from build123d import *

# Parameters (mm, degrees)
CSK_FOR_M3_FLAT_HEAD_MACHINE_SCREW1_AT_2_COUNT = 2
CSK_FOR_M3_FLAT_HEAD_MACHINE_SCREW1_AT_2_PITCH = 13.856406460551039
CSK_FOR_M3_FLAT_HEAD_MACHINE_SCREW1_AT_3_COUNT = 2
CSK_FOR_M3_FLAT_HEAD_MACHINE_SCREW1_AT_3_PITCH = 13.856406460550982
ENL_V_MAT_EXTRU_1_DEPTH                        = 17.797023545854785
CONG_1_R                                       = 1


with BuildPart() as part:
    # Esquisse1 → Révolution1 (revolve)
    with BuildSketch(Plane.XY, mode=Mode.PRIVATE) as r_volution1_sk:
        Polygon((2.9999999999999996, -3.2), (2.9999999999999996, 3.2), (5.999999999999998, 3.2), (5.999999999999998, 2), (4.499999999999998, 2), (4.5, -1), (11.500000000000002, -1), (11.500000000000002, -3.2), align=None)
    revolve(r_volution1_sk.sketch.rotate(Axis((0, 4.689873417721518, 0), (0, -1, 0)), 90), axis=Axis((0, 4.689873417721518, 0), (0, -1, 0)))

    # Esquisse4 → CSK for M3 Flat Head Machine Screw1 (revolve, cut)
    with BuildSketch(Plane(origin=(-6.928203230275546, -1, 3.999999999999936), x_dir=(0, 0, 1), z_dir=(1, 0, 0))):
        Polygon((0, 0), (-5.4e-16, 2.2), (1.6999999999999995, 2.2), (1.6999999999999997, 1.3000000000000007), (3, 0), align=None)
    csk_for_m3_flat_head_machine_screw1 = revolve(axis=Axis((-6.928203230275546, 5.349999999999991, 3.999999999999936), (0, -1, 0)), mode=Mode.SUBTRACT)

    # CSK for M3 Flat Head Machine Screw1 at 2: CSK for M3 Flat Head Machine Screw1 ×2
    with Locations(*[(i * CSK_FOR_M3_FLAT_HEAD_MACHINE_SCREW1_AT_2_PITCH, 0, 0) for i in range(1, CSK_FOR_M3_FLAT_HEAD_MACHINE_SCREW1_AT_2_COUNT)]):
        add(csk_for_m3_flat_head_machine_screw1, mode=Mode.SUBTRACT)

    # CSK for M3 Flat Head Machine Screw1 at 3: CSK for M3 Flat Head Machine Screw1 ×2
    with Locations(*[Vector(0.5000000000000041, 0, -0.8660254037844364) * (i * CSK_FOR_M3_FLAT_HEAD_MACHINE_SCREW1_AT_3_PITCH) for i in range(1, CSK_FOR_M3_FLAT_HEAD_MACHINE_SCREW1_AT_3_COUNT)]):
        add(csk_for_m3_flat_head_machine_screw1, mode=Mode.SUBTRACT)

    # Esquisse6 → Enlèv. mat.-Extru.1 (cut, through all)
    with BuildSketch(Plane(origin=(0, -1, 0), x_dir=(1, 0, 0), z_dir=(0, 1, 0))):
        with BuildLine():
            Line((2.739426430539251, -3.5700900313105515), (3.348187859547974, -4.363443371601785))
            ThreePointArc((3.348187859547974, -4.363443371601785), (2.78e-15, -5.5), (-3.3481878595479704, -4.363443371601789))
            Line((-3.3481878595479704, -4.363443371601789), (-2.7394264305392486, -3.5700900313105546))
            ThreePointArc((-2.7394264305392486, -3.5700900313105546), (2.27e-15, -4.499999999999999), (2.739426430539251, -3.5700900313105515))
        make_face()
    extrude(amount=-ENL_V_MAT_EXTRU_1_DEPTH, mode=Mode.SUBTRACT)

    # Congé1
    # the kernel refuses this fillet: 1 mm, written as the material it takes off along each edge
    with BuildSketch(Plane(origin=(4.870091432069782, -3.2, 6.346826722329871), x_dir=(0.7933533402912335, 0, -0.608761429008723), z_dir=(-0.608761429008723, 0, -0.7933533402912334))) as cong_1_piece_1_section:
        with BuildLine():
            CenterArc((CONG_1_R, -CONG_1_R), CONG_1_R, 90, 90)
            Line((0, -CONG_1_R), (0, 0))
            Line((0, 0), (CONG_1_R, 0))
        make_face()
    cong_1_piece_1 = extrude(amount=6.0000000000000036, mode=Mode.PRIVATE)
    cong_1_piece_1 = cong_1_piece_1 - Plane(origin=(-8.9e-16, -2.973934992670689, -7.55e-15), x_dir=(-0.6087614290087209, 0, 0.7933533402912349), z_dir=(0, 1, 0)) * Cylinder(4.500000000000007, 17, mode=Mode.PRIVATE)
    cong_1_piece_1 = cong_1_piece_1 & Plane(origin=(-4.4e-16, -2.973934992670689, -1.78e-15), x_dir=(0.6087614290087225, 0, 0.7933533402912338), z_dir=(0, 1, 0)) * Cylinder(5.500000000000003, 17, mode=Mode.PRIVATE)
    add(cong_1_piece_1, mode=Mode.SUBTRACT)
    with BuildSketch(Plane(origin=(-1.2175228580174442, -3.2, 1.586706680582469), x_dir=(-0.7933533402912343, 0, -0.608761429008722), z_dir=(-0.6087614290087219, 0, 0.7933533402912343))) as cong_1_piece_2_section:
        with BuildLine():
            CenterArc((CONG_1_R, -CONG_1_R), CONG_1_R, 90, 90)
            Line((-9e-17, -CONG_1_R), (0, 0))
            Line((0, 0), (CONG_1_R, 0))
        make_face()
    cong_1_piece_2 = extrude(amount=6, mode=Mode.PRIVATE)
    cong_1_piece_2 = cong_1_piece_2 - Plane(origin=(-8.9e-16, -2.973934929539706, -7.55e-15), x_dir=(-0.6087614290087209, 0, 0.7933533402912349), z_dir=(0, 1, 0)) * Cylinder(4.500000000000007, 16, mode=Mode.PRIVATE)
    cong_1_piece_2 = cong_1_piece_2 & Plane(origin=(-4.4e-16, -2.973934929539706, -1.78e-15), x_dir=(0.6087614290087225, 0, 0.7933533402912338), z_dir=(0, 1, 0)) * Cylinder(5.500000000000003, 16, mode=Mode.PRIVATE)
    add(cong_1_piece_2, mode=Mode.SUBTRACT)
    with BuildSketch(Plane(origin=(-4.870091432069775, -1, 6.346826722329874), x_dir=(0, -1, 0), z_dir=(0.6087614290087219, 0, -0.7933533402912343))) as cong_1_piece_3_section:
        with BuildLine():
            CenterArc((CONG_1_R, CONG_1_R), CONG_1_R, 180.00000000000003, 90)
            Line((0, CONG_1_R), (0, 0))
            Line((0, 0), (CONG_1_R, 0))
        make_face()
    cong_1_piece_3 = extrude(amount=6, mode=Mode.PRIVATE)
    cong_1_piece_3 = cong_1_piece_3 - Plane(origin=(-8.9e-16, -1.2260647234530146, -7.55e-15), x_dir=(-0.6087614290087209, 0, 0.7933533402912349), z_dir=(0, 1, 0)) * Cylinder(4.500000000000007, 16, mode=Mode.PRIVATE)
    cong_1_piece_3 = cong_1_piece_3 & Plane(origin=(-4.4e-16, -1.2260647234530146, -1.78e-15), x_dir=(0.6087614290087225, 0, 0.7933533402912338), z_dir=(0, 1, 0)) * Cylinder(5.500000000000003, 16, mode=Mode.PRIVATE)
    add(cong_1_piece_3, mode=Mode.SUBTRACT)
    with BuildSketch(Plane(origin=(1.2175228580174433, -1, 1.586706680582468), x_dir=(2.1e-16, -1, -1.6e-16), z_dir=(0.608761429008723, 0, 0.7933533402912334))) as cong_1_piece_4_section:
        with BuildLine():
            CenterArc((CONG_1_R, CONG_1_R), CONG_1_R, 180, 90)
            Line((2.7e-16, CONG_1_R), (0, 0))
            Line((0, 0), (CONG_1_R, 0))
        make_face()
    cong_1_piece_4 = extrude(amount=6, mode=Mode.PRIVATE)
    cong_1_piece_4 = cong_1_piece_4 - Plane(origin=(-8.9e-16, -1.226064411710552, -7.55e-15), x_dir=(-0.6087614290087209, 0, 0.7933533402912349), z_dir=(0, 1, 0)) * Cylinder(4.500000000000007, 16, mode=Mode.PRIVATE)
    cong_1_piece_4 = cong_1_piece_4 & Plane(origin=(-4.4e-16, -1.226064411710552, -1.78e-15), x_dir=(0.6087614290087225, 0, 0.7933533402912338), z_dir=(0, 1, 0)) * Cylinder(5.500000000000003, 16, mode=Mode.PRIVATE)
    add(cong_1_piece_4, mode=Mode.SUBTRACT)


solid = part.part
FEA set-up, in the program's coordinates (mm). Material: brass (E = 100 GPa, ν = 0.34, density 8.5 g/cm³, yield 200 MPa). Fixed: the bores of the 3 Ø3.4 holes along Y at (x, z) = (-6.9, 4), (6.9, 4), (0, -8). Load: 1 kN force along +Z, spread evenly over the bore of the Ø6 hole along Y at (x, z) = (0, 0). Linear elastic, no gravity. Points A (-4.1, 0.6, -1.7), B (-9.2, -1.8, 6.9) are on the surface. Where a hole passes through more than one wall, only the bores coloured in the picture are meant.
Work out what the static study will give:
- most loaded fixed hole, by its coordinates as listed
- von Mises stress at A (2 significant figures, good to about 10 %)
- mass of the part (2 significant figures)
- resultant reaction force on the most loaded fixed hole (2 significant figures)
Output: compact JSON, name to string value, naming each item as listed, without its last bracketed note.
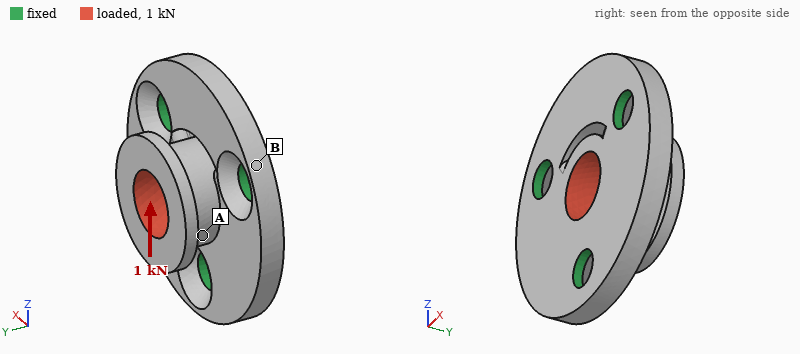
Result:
{"most loaded fixed hole, by its coordinates as listed": "(0, -8)", "von Mises stress at A": "35 MPa", "mass of the part": "8.1 g", "resultant reaction force on the most loaded fixed hole": "490 N"}
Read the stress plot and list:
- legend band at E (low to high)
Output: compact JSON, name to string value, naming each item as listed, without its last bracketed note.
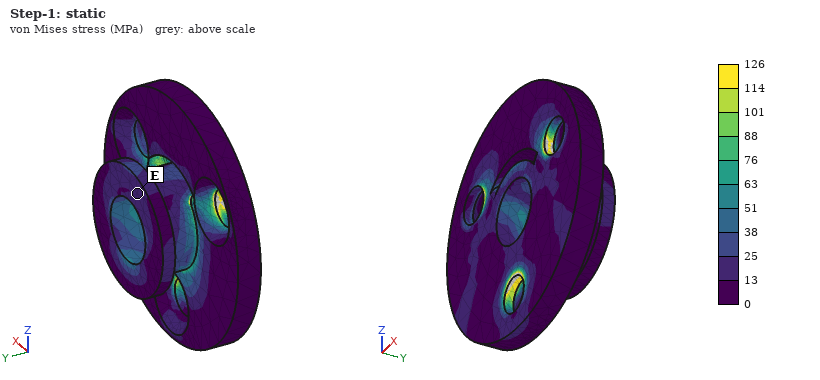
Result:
{"legend band at E": "13 to 25 MPa"}
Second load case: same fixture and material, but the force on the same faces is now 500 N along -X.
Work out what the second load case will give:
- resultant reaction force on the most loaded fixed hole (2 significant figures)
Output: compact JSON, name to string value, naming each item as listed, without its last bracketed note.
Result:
{"resultant reaction force on the most loaded fixed hole": "200 N"}
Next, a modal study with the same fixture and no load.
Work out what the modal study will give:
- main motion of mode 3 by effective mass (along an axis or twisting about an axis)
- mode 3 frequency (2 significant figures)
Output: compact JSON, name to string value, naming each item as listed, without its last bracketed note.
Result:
{"main motion of mode 3 by effective mass": "along Y", "mode 3 frequency": "20 kHz"}
